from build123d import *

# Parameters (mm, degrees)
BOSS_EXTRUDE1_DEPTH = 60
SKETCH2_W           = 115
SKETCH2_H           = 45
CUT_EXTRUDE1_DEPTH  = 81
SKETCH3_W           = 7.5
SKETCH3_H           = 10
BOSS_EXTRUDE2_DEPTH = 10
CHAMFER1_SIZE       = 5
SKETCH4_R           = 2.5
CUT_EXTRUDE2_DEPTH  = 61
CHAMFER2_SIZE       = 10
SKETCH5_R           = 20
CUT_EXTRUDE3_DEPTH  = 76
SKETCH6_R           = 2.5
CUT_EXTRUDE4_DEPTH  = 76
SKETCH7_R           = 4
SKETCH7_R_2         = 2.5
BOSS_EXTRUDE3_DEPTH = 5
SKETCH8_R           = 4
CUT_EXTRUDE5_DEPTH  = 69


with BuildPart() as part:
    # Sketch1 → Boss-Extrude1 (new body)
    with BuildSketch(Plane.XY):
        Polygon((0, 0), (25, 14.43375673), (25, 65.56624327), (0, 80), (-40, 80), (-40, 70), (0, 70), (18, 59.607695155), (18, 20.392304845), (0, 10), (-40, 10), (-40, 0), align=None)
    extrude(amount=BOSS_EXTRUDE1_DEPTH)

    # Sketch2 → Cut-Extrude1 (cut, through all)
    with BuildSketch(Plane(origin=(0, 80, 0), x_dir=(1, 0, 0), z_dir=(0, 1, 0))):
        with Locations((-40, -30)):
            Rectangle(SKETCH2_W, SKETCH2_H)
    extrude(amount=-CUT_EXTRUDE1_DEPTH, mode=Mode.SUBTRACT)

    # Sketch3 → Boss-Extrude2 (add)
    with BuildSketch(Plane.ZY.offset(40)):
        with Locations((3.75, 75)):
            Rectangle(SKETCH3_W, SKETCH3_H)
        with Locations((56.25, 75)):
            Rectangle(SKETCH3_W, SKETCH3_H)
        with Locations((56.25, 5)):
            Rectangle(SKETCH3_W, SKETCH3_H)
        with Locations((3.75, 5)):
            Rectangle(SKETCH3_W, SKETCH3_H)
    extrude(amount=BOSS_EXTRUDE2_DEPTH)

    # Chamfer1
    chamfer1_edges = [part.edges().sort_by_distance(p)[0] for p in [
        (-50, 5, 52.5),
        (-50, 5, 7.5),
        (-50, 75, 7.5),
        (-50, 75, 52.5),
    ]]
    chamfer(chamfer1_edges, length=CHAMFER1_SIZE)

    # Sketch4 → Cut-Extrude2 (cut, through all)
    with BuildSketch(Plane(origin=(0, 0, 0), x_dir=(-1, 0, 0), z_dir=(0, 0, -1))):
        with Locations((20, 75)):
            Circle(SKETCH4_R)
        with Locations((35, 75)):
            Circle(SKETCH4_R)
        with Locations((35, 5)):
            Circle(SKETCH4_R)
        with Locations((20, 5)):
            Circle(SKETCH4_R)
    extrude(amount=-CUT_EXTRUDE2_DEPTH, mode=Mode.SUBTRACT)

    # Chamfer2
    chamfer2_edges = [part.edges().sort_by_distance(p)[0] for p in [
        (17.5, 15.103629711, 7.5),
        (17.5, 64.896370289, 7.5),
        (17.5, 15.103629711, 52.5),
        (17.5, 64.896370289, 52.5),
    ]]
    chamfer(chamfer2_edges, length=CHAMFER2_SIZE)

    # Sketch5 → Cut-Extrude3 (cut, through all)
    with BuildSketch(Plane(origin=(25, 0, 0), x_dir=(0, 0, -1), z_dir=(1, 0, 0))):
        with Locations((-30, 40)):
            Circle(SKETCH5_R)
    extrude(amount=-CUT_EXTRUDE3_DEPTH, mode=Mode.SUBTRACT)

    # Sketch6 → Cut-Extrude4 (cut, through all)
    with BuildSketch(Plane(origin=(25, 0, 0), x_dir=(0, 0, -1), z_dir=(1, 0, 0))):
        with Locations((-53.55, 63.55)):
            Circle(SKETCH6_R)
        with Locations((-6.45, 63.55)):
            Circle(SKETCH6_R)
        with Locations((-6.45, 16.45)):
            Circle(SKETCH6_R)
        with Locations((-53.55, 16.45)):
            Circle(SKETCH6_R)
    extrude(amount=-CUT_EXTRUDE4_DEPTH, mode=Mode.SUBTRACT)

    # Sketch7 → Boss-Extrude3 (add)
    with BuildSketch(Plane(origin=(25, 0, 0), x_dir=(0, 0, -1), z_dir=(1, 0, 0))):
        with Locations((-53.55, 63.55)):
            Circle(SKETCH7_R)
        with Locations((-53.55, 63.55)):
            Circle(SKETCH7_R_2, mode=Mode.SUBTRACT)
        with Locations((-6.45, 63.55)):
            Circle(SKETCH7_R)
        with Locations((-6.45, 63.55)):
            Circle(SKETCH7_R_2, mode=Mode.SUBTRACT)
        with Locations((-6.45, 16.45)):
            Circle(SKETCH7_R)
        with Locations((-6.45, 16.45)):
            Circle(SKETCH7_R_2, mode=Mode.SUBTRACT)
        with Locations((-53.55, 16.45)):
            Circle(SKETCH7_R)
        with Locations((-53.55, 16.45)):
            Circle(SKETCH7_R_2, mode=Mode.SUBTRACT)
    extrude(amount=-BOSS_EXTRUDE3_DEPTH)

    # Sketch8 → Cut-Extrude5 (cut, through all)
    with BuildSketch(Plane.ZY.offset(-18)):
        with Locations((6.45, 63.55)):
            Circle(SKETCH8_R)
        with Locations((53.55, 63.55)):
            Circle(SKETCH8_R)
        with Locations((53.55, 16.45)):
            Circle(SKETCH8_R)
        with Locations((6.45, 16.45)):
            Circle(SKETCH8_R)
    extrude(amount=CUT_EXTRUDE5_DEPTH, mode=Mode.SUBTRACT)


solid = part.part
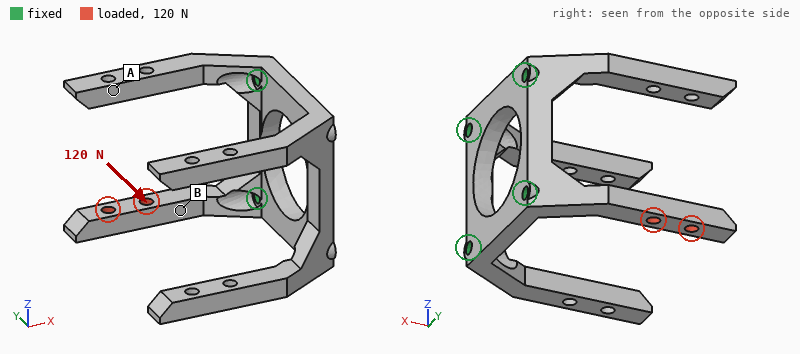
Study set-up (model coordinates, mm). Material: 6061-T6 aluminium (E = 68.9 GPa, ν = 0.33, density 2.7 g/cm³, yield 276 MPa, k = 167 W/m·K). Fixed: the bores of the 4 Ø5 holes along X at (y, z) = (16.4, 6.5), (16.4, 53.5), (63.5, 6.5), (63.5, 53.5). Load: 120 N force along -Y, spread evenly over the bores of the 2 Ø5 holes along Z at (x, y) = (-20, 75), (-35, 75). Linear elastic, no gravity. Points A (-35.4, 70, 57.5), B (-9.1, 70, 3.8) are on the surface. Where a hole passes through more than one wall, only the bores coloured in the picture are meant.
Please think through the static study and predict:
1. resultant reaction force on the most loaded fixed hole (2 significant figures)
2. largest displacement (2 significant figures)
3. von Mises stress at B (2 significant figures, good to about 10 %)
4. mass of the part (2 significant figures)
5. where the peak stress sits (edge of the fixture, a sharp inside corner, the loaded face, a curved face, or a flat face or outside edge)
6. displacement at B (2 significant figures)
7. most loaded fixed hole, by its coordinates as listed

110 N
0.34 mm
17 MPa
91 g
a curved face
0.10 mm
(63.5, 6.5)
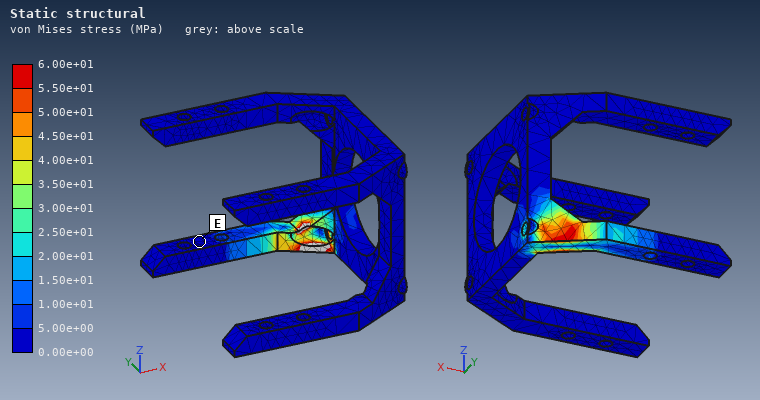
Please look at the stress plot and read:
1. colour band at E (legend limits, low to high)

0.00e+00 to 5.00e+00 MPa
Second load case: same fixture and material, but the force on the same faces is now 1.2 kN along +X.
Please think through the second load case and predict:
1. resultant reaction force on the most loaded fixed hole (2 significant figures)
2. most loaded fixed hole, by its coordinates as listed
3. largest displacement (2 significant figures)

1.3 kN
(63.5, 6.5)
0.47 mm
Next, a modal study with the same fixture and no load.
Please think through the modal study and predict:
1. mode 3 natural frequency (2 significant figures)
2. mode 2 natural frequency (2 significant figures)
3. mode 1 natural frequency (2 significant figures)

1200 Hz
1200 Hz
1200 Hz
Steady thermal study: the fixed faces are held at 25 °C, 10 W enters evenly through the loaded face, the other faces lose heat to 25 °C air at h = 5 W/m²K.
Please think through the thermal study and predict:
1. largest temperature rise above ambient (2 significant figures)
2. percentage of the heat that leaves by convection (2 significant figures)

45 K
3.6 %
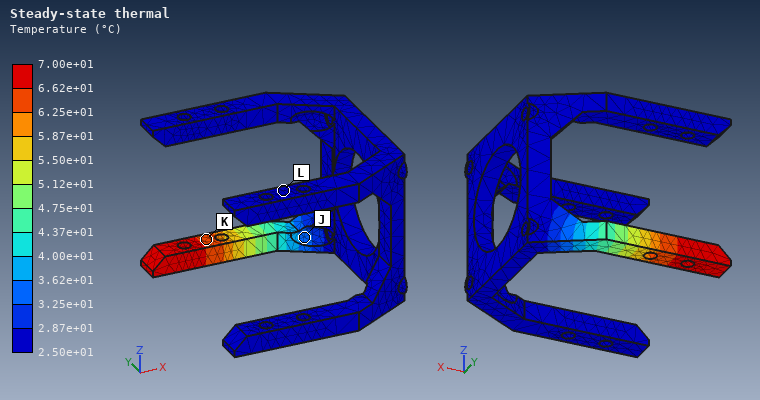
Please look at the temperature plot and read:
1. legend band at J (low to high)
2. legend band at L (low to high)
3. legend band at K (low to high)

3.25e+01 to 3.62e+01 °C
2.50e+01 to 2.87e+01 °C
6.25e+01 to 6.62e+01 °C
